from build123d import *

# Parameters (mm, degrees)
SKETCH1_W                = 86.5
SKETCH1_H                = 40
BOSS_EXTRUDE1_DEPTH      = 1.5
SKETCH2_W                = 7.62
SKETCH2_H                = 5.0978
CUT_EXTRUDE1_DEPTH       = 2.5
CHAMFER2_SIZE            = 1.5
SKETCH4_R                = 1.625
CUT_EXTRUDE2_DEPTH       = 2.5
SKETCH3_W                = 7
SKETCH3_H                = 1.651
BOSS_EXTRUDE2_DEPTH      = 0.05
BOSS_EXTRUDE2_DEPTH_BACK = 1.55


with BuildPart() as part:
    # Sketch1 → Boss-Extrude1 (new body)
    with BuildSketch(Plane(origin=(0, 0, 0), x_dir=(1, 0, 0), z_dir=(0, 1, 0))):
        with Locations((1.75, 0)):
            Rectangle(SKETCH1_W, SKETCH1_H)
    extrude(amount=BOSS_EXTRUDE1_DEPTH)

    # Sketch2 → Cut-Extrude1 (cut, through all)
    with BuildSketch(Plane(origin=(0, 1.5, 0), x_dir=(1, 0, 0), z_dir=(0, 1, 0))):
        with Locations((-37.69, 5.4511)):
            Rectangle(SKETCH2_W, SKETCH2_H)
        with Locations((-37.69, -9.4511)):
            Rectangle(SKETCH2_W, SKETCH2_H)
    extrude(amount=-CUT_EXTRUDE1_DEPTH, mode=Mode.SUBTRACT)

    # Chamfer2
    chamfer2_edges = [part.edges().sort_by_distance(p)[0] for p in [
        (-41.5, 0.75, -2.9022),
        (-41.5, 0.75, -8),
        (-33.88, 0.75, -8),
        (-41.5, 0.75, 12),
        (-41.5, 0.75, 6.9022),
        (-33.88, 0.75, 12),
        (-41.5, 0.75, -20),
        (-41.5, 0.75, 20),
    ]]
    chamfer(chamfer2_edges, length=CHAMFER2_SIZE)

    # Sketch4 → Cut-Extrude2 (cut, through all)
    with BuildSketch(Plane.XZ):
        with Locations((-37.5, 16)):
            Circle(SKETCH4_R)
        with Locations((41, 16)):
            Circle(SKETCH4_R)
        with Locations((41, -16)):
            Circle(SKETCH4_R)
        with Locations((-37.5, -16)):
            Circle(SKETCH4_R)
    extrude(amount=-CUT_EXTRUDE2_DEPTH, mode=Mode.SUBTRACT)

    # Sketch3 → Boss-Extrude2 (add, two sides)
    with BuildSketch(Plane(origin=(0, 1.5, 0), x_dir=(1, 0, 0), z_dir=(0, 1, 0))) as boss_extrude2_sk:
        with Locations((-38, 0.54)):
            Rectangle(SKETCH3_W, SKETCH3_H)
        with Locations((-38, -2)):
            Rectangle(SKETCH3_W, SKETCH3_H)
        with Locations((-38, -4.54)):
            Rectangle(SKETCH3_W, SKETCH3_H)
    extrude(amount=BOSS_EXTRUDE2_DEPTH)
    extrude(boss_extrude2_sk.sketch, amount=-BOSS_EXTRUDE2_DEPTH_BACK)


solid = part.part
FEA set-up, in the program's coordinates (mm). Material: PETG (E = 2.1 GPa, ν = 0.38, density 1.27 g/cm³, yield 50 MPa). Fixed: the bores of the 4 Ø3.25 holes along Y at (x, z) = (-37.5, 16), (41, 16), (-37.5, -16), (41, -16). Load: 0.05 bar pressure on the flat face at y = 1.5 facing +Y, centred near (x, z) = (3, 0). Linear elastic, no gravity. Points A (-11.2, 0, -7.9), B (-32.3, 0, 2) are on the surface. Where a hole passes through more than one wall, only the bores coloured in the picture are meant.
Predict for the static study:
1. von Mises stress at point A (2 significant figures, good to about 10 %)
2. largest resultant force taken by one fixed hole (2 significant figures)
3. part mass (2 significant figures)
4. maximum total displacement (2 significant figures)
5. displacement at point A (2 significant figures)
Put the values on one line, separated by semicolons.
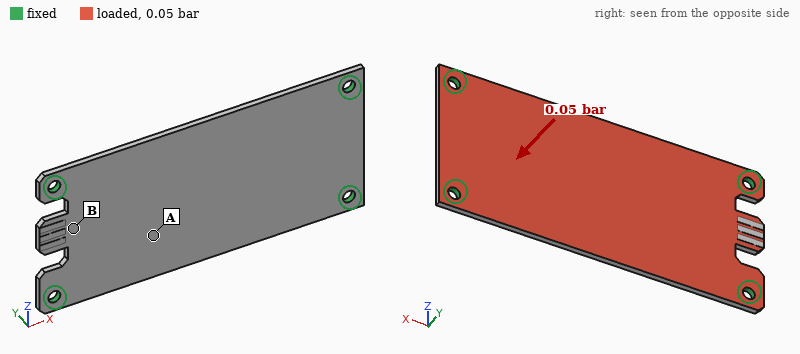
2.5 MPa; 4.4 N; 6.4 g; 1.00 mm; 0.76 mm
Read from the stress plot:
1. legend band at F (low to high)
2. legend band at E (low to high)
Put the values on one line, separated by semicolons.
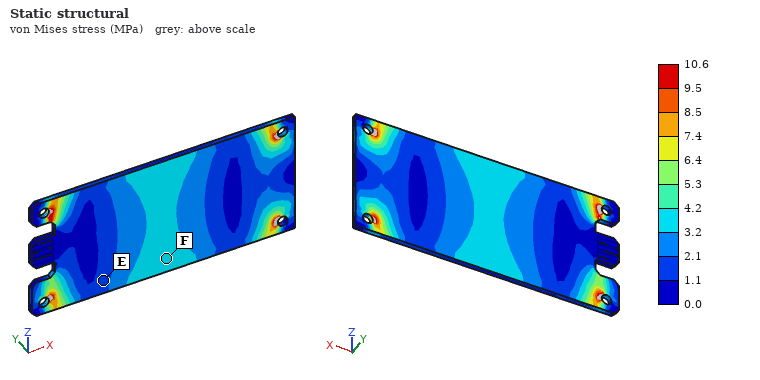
3.2 to 4.2 MPa; 1.1 to 2.1 MPa
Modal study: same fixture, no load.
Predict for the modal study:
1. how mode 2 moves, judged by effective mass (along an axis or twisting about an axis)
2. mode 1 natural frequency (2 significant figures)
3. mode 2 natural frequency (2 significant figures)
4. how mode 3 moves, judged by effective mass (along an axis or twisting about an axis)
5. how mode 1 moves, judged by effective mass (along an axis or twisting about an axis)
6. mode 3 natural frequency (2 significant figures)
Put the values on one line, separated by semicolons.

twisting about X; 300 Hz; 540 Hz; twisting about Z; along Y; 850 Hz
